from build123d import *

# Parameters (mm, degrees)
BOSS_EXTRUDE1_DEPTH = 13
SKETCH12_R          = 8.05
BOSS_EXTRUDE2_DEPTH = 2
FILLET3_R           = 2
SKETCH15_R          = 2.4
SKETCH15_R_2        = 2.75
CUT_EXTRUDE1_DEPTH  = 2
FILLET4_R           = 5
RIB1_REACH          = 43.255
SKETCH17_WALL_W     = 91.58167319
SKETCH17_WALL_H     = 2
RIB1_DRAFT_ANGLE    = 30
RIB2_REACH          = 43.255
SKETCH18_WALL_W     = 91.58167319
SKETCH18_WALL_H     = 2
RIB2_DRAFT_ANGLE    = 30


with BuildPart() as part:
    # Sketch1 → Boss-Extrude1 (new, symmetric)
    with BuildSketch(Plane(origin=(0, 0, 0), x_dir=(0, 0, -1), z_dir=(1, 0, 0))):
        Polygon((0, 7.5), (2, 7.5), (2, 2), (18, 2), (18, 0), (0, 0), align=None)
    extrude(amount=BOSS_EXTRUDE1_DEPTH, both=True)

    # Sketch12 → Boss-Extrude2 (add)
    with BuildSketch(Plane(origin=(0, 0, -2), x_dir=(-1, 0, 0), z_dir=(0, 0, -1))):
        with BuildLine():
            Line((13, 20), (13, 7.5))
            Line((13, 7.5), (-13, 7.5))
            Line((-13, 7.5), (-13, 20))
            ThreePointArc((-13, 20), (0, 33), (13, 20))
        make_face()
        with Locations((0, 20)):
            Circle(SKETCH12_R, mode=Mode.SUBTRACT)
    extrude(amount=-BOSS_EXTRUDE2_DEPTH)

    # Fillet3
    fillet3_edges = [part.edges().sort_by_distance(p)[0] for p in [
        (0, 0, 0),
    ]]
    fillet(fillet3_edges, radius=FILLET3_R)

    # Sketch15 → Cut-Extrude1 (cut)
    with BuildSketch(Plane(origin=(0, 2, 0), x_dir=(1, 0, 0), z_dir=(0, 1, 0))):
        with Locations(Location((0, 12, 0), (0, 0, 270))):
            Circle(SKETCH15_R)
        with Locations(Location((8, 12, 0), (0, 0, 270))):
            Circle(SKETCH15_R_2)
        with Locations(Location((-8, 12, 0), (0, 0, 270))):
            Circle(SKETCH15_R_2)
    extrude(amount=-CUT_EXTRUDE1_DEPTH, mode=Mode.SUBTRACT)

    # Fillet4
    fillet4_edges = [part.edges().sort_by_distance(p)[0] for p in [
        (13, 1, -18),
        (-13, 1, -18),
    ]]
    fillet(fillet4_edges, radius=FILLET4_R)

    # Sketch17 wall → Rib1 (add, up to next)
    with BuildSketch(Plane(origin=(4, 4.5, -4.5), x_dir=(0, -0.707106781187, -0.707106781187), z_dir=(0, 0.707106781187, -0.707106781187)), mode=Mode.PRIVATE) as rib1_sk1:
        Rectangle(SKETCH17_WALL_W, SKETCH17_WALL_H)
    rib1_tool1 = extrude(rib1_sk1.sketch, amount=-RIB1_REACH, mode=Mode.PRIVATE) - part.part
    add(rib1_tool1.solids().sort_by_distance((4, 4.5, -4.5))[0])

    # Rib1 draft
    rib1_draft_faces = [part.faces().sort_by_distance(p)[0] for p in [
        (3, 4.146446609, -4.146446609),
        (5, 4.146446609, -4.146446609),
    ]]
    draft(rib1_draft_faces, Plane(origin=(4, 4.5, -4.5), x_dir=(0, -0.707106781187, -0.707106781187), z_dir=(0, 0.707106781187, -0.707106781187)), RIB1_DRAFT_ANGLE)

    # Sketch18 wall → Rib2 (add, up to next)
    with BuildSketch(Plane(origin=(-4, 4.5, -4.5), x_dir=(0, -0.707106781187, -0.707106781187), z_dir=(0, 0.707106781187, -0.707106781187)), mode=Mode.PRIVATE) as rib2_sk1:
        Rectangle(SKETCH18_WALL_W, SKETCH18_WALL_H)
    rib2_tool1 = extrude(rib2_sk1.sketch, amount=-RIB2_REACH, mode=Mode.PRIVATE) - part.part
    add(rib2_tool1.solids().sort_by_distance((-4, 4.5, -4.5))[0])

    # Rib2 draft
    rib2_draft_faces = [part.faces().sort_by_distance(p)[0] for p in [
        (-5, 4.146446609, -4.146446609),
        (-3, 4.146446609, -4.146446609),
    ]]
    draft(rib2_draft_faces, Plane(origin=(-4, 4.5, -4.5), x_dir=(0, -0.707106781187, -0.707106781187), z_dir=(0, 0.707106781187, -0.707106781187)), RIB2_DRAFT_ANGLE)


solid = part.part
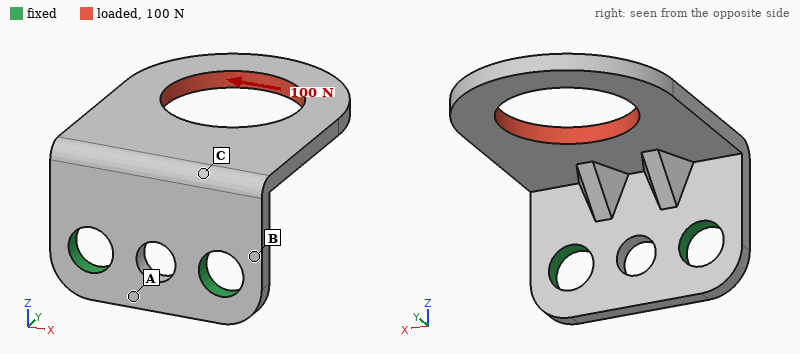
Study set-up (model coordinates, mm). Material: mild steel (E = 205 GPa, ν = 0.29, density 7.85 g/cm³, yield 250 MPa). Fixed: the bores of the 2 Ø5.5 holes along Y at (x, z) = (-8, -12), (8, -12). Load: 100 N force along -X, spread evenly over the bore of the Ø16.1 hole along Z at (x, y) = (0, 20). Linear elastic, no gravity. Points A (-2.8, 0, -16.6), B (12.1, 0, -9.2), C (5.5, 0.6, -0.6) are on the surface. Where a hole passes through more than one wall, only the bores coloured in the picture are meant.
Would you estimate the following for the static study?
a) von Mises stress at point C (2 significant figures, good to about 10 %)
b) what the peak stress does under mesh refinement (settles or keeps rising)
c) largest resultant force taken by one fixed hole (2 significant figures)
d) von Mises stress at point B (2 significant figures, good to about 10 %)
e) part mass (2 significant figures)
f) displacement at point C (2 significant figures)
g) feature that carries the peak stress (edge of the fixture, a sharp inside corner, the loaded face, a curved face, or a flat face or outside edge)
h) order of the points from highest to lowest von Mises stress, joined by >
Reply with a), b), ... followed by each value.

a) 17 MPa
b) keeps rising
c) 130 N
d) 39 MPa
e) 15 g
f) 3.6 µm
g) edge of the fixture
h) B > C > A
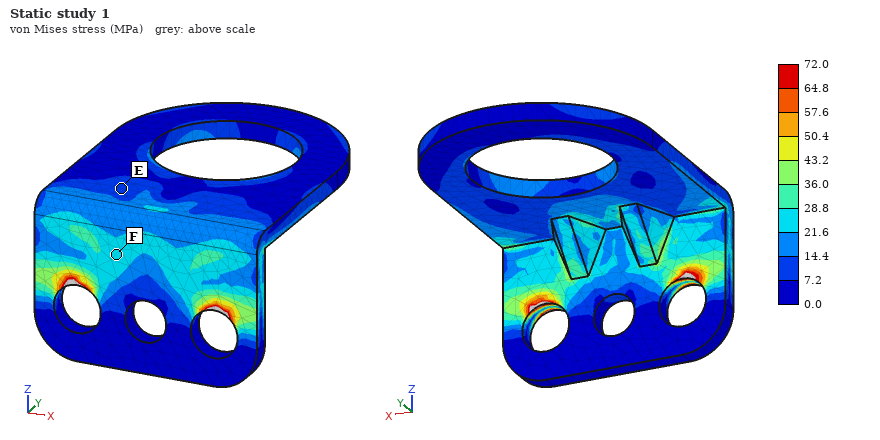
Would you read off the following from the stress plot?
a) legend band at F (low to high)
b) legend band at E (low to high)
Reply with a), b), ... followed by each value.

a) 21.6 to 28.8 MPa
b) 7.2 to 14.4 MPa
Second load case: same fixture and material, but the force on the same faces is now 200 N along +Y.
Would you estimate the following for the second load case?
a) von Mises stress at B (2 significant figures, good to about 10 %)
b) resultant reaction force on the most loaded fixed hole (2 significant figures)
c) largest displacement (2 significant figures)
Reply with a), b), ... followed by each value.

a) 64 MPa
b) 100 N
c) 65 µm
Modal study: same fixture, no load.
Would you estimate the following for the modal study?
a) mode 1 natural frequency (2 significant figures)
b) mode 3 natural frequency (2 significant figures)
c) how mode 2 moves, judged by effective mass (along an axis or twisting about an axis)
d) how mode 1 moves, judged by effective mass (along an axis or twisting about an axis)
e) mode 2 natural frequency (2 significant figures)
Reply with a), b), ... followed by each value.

a) 1800 Hz
b) 5700 Hz
c) along X
d) along Z
e) 4400 Hz
